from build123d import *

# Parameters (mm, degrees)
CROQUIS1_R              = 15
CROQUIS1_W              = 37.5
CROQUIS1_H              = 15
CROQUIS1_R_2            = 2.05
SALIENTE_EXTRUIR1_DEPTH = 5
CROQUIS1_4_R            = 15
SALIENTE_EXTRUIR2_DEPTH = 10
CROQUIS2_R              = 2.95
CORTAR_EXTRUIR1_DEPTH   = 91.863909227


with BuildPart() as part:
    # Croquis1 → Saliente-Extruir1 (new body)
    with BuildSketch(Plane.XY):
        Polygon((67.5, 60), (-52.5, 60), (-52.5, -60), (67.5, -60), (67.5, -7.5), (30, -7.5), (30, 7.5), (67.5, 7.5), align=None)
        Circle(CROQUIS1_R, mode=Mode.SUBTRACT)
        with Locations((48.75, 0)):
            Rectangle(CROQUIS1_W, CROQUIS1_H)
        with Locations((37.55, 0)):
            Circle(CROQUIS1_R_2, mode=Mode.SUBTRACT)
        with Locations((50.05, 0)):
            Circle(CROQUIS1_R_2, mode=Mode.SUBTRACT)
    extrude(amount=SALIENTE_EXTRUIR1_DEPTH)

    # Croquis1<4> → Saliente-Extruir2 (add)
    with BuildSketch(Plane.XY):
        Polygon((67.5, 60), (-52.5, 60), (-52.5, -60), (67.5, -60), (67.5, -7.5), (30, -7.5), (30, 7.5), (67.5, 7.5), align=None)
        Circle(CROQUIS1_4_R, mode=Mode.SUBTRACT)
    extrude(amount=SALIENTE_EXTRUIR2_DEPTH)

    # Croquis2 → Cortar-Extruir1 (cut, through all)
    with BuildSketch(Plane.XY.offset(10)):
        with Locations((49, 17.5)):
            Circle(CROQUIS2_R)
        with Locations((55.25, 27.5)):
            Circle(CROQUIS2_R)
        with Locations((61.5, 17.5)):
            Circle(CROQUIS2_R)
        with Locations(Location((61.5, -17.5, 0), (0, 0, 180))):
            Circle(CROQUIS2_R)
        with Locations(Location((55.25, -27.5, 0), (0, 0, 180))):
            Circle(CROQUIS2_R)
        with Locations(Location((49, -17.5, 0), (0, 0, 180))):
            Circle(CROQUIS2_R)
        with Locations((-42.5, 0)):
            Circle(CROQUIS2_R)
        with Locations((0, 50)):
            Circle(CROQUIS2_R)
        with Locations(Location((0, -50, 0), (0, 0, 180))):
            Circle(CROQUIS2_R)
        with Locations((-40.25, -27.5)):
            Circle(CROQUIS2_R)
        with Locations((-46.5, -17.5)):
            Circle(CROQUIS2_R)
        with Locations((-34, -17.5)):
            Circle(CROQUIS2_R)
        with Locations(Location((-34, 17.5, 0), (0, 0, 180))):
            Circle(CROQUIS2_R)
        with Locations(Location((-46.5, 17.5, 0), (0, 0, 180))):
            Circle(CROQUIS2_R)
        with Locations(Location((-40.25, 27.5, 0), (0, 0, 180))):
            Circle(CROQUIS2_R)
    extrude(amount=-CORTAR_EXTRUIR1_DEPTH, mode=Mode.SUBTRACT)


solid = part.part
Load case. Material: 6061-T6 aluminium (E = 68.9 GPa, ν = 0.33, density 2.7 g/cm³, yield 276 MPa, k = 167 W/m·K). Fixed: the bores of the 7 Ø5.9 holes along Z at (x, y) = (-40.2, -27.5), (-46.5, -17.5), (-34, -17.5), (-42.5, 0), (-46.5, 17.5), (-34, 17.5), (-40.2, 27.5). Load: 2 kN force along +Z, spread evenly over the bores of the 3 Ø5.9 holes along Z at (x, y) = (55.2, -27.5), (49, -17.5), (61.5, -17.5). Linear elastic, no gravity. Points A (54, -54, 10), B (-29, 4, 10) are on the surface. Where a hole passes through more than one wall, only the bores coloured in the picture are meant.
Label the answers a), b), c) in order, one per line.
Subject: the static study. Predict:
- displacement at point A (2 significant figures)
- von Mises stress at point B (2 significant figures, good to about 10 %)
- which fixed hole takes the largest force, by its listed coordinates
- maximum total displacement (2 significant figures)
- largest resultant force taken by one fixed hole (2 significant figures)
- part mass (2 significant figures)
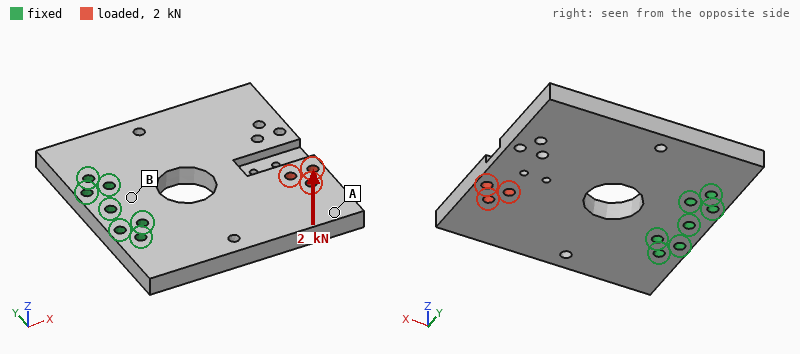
a) 1.1 mm
b) 55 MPa
c) (-34, -17.5)
d) 1.3 mm
e) 3.3 kN
f) 350 g
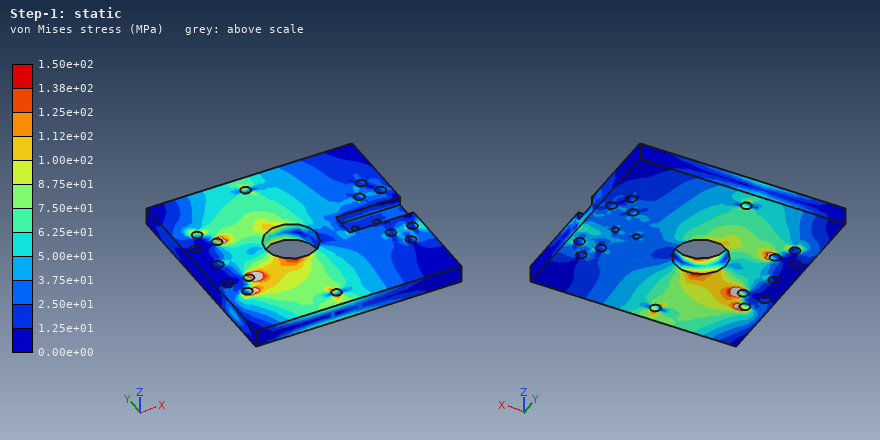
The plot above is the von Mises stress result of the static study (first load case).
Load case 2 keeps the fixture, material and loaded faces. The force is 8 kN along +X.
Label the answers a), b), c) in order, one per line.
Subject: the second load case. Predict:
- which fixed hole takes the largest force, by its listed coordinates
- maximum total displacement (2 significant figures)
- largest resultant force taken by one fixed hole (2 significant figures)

a) (-40.2, -27.5)
b) 37 µm
c) 4.5 kN
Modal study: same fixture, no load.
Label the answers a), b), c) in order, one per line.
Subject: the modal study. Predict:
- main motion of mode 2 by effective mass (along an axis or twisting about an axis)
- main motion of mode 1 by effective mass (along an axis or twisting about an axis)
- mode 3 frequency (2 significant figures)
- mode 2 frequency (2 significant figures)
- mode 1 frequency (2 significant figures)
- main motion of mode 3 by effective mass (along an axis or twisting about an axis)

a) twisting about X
b) along Z
c) 3200 Hz
d) 1300 Hz
e) 710 Hz
f) along Y
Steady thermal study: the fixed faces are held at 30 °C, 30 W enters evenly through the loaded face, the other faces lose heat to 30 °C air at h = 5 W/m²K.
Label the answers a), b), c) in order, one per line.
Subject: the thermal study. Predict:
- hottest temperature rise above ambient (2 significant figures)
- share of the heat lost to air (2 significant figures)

a) 25 K
b) 4.9 %
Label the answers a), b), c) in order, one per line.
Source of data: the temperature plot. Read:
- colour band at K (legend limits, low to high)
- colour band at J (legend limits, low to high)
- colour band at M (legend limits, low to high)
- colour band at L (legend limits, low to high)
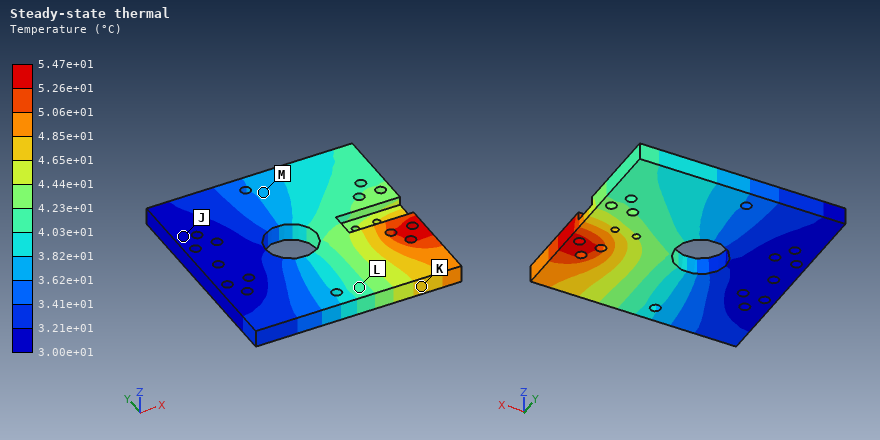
a) 4.65e+01 to 4.85e+01 °C
b) 3.00e+01 to 3.21e+01 °C
c) 3.62e+01 to 3.82e+01 °C
d) 4.03e+01 to 4.23e+01 °C
